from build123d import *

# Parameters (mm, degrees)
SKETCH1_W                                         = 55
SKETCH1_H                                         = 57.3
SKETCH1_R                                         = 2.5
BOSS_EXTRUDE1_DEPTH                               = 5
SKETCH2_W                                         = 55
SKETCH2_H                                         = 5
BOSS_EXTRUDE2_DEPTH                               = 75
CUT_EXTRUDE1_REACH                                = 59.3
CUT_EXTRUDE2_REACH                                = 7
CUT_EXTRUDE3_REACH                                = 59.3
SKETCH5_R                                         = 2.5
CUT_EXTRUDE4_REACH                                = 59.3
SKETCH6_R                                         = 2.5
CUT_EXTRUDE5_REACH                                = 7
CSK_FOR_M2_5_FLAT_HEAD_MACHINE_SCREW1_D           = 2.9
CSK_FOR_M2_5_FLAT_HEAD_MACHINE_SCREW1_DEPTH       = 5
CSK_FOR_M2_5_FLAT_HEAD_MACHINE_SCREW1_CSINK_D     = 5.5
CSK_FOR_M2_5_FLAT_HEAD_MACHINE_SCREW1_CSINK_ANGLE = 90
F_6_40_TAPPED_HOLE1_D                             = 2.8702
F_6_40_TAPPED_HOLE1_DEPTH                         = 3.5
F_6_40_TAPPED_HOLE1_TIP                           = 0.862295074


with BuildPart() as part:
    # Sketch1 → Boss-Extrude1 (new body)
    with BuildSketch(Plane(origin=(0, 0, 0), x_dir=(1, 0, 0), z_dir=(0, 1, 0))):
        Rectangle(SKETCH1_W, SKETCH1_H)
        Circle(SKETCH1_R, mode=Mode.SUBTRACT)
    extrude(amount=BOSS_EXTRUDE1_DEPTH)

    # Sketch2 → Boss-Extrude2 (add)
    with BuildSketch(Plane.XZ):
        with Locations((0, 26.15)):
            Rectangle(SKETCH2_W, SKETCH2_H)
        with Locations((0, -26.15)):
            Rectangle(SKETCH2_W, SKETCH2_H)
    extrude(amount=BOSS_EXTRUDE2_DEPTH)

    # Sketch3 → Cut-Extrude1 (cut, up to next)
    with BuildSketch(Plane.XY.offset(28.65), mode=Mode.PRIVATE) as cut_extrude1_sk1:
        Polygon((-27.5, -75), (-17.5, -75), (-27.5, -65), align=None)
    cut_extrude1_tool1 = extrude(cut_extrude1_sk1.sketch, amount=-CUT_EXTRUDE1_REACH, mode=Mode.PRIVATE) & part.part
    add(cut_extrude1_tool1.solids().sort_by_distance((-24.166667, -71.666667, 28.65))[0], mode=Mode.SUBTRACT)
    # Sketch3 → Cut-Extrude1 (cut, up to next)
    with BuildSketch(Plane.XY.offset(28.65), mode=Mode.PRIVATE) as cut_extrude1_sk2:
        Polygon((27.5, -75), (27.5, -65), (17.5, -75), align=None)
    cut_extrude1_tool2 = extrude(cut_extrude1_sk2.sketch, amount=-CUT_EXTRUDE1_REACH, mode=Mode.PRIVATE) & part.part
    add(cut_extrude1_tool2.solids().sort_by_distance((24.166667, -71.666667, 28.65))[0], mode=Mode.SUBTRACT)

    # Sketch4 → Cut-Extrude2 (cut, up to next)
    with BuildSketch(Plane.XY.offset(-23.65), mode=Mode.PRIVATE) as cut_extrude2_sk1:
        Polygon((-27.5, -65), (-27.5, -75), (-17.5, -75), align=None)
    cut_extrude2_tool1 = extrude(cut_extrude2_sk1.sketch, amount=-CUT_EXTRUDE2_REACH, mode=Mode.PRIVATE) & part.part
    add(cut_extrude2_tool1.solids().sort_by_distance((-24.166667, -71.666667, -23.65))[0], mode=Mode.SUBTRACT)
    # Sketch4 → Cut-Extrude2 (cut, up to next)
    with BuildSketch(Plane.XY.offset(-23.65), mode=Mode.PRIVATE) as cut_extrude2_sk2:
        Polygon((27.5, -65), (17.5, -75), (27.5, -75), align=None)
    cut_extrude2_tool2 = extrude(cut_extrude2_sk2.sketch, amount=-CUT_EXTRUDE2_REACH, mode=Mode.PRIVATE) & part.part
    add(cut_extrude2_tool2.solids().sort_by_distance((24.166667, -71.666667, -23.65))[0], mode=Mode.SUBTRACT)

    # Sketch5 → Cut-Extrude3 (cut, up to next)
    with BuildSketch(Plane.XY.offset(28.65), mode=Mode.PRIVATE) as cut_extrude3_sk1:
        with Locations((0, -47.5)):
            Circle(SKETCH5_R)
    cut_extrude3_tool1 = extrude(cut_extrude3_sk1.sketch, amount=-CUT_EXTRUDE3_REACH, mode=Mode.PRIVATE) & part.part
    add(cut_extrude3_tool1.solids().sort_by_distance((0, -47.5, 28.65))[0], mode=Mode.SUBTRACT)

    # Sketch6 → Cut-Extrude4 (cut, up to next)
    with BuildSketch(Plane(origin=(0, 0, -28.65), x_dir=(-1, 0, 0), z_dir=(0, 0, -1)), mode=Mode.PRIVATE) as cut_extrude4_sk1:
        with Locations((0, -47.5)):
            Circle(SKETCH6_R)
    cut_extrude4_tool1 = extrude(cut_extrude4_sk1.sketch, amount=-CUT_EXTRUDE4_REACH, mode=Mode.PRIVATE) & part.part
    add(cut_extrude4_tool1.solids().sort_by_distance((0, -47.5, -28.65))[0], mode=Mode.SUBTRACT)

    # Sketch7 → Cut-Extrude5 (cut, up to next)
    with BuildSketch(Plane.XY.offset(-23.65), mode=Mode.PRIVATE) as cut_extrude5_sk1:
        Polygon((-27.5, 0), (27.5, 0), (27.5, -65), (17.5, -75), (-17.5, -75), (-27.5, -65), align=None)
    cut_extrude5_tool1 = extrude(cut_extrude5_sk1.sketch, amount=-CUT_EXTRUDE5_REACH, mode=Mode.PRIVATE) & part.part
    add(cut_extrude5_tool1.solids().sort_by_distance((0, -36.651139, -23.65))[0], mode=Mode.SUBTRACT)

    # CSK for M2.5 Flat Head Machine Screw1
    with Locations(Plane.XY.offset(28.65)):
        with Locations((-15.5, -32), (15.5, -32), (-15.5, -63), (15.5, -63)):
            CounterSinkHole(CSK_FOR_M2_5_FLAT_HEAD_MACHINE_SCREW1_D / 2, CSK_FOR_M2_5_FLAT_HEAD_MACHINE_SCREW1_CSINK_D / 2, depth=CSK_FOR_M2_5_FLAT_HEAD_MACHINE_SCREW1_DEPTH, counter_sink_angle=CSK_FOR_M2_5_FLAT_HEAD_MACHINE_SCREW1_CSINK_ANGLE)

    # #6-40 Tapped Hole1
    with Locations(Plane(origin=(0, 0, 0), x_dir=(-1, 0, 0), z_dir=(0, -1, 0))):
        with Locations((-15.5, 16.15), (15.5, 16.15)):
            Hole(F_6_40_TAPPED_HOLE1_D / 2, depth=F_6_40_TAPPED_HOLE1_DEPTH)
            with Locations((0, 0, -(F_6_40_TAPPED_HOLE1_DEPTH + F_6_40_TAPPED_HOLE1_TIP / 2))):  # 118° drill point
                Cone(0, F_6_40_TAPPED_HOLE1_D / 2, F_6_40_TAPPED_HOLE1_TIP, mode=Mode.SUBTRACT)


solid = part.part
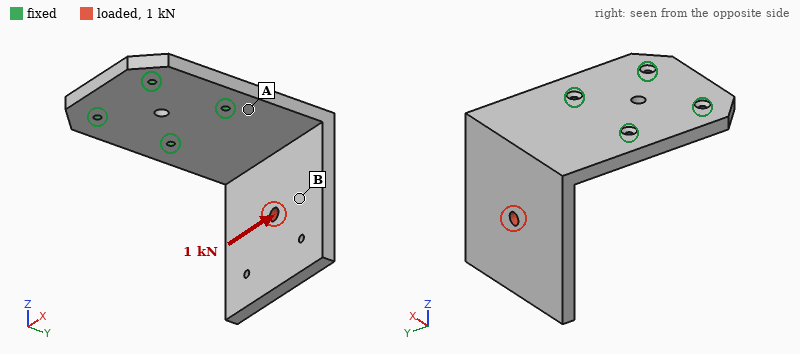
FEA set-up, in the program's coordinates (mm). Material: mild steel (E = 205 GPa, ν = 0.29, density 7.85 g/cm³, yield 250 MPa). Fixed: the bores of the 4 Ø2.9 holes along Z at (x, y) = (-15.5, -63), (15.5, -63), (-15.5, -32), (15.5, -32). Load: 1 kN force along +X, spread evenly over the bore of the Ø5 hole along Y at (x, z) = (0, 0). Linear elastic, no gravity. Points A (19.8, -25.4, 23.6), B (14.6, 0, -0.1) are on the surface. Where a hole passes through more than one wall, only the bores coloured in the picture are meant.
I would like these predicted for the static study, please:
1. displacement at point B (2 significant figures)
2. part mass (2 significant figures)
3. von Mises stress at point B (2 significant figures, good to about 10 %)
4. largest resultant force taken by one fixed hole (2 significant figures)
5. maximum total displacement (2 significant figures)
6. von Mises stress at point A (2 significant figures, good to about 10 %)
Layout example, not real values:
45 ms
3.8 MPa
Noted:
0.094 mm
280 g
12 MPa
1.2 kN
0.19 mm
61 MPa
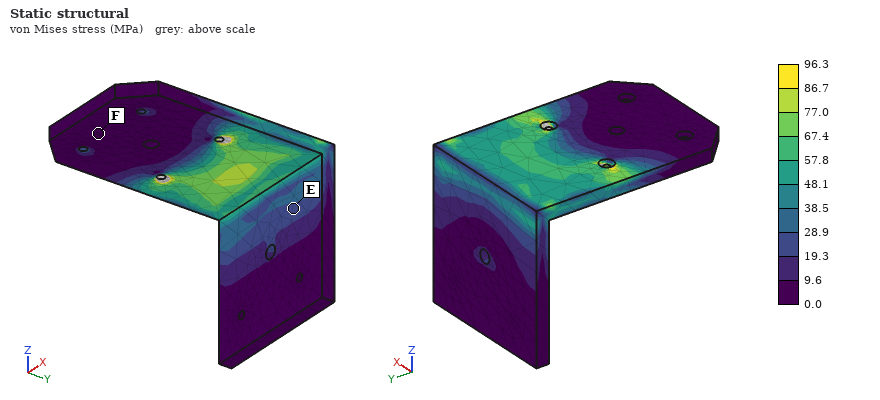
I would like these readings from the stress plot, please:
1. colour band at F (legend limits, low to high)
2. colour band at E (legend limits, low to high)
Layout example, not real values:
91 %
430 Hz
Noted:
0.0 to 9.6 MPa
19.3 to 28.9 MPa
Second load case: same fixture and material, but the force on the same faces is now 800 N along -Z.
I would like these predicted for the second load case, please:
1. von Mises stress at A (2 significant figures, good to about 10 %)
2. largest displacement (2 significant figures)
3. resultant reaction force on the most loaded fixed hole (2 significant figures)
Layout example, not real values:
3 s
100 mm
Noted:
95 MPa
0.29 mm
690 N
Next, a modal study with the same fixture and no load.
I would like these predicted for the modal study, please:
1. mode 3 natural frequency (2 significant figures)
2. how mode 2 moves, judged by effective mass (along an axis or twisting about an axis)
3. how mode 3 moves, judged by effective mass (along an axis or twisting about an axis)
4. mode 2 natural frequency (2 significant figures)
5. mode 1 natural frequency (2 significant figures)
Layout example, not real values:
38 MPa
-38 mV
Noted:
1900 Hz
along X
along Z
1200 Hz
650 Hz
